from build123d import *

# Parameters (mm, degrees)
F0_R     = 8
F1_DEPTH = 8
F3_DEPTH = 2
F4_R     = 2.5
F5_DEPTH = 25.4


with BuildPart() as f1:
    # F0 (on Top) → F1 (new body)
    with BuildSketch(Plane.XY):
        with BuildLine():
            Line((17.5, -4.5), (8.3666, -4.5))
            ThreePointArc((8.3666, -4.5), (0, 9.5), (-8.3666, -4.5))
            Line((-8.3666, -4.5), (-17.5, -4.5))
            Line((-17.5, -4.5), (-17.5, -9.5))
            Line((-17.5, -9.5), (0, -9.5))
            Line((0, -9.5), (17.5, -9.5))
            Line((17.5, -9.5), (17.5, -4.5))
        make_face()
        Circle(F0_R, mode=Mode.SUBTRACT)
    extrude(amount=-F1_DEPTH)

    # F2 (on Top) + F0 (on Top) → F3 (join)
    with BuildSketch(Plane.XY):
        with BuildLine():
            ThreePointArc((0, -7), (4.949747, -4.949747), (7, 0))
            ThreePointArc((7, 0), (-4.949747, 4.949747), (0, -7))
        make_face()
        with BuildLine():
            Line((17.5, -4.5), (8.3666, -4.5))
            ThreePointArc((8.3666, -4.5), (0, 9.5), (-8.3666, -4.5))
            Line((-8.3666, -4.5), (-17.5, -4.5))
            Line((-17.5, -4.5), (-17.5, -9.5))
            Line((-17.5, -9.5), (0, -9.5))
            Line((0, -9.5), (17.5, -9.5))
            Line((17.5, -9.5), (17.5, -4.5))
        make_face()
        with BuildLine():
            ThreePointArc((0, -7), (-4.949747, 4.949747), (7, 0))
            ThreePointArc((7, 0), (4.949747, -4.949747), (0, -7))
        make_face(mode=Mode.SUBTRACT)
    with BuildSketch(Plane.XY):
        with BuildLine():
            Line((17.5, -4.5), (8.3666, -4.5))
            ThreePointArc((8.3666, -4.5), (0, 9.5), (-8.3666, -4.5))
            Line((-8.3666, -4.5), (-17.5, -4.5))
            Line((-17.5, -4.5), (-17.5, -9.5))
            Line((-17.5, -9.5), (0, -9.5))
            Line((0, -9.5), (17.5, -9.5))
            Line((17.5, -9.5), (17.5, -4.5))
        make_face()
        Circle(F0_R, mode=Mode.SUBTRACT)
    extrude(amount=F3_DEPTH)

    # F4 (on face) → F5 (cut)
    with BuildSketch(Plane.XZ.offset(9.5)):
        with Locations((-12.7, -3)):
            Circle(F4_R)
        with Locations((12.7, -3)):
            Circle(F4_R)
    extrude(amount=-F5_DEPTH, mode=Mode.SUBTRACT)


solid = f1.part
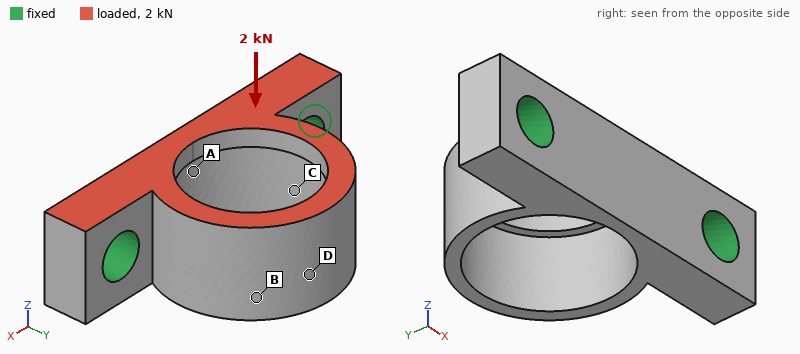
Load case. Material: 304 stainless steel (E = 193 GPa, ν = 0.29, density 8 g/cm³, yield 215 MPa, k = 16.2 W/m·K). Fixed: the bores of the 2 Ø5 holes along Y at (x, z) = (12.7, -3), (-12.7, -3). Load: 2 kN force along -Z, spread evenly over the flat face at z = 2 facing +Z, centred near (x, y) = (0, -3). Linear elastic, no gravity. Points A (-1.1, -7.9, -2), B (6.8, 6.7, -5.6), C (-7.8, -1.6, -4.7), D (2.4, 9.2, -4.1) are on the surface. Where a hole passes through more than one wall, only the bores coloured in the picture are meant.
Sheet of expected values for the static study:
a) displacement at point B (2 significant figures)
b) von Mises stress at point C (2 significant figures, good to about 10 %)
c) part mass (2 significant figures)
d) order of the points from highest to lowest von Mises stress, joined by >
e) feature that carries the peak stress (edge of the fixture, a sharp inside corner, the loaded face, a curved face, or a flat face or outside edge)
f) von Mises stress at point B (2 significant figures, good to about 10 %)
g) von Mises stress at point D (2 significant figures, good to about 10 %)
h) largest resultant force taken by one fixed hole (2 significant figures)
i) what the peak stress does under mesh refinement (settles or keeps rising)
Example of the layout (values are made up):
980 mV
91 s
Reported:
20 µm
110 MPa
15 g
C > B > D > A
a sharp inside corner
54 MPa
28 MPa
1.0 kN
keeps rising
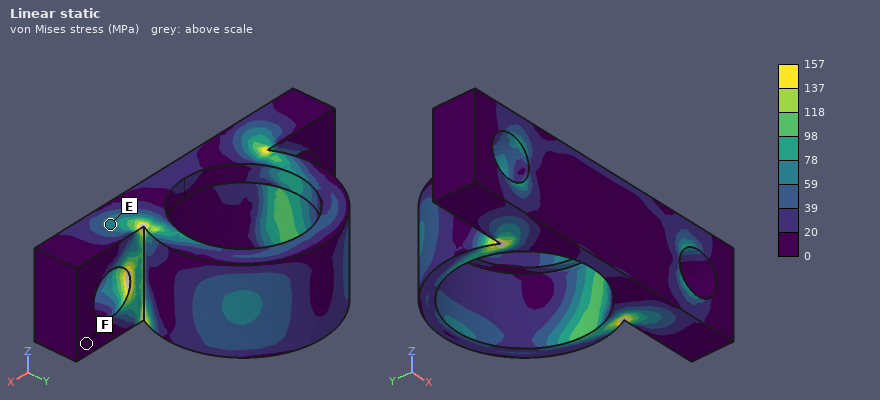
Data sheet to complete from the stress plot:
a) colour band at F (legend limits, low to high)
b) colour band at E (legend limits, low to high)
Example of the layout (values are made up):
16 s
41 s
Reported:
0 to 20 MPa
59 to 78 MPa
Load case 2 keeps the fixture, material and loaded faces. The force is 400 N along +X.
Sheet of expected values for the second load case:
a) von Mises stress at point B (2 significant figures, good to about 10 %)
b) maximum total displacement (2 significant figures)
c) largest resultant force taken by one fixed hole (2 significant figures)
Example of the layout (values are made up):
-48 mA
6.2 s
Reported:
16 MPa
8.9 µm
210 N
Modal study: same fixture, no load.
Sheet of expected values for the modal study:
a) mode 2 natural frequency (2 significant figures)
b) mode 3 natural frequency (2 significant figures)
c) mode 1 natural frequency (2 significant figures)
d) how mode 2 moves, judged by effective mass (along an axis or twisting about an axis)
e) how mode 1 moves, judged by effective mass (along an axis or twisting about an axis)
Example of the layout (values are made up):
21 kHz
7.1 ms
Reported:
13 kHz
23 kHz
9700 Hz
along Z
along X
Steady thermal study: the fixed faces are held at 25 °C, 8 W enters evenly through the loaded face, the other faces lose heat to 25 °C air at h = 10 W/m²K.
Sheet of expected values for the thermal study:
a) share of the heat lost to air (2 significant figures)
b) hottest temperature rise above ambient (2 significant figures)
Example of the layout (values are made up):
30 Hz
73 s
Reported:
5.1 %
63 K
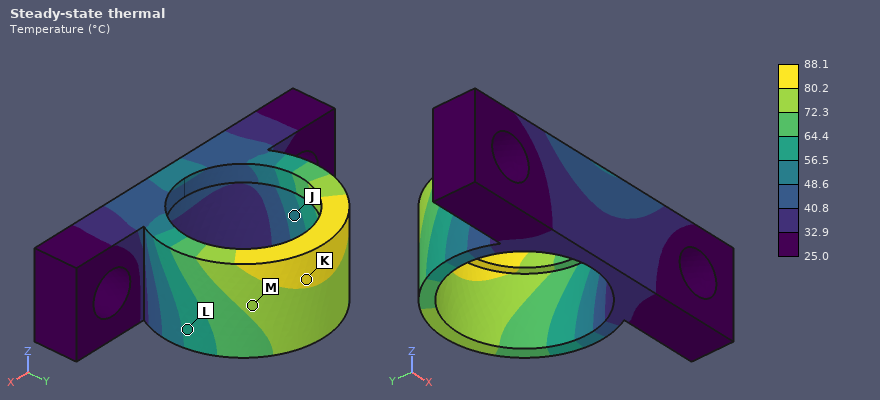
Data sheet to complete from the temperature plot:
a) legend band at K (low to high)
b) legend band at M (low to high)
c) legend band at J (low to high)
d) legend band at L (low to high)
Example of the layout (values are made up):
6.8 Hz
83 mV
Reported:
80.2 to 88.1 °C
72.3 to 80.2 °C
48.6 to 56.5 °C
56.5 to 64.4 °C
